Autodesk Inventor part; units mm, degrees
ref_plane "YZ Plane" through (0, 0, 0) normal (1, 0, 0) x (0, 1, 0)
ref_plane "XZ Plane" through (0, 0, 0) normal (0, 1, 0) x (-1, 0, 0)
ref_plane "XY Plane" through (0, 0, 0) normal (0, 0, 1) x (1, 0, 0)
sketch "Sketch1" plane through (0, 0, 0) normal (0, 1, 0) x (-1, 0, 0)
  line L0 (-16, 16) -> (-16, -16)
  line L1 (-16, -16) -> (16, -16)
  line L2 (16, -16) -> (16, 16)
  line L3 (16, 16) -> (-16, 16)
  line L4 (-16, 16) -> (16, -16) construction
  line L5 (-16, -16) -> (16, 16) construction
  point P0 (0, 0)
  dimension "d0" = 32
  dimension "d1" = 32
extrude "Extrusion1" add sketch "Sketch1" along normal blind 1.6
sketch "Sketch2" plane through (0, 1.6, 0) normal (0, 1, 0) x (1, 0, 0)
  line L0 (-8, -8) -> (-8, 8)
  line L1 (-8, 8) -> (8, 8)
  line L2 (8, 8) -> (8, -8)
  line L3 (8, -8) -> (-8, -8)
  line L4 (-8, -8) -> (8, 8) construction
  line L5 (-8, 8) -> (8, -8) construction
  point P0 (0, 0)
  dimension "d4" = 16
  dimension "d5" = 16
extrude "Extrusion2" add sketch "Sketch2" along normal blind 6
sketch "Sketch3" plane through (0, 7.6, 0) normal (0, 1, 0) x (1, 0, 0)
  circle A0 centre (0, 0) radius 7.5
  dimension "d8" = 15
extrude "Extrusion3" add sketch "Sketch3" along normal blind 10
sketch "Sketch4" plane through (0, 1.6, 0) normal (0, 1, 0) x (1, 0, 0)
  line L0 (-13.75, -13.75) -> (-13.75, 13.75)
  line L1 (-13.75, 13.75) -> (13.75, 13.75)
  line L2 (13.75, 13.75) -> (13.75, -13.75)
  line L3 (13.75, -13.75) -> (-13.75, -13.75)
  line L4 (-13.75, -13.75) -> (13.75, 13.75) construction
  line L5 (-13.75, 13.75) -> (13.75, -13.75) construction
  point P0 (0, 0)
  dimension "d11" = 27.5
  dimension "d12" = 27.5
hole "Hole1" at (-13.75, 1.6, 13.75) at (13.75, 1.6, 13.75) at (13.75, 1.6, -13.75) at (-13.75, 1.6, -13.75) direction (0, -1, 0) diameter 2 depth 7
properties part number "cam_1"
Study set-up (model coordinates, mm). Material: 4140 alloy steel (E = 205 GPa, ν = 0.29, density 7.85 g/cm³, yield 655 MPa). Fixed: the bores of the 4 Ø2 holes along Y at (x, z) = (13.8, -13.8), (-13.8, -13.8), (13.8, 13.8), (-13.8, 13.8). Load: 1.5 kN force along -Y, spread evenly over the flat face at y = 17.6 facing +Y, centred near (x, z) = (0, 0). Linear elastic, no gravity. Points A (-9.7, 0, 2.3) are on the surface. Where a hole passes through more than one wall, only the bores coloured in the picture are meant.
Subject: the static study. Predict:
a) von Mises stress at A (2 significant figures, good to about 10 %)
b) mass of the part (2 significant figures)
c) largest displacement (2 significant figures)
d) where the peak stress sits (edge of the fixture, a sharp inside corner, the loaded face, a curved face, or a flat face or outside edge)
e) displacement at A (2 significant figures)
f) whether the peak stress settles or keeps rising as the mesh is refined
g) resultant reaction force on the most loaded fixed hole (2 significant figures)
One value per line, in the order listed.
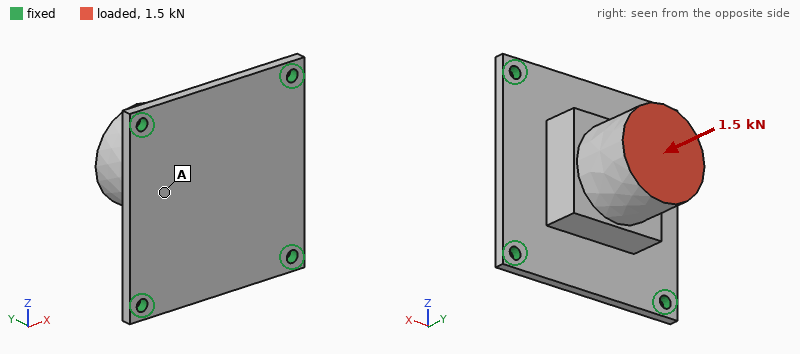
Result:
99 MPa
39 g
45 µm
edge of the fixture
43 µm
keeps rising
400 N
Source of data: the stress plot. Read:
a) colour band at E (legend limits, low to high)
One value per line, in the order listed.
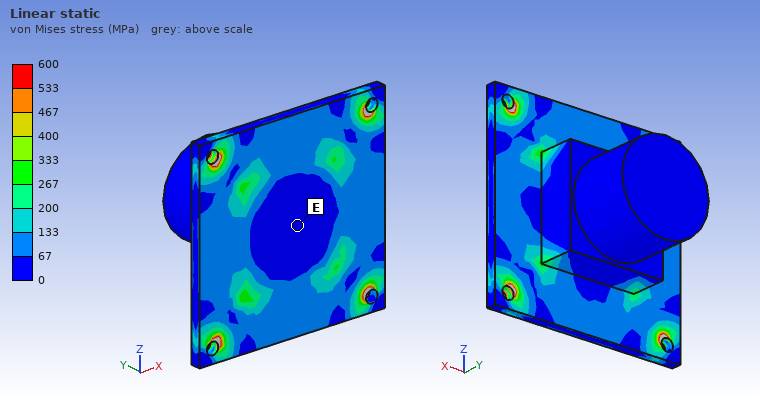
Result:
0 to 67 MPa
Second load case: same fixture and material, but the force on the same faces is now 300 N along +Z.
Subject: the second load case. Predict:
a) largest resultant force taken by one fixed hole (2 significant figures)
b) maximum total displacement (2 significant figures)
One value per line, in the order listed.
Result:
140 N
23 µm
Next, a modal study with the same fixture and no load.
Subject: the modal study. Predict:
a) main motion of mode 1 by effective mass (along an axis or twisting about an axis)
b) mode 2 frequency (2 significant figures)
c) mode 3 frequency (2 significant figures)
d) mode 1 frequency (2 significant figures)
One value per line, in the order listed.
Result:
along Y
5800 Hz
5800 Hz
5000 Hz
